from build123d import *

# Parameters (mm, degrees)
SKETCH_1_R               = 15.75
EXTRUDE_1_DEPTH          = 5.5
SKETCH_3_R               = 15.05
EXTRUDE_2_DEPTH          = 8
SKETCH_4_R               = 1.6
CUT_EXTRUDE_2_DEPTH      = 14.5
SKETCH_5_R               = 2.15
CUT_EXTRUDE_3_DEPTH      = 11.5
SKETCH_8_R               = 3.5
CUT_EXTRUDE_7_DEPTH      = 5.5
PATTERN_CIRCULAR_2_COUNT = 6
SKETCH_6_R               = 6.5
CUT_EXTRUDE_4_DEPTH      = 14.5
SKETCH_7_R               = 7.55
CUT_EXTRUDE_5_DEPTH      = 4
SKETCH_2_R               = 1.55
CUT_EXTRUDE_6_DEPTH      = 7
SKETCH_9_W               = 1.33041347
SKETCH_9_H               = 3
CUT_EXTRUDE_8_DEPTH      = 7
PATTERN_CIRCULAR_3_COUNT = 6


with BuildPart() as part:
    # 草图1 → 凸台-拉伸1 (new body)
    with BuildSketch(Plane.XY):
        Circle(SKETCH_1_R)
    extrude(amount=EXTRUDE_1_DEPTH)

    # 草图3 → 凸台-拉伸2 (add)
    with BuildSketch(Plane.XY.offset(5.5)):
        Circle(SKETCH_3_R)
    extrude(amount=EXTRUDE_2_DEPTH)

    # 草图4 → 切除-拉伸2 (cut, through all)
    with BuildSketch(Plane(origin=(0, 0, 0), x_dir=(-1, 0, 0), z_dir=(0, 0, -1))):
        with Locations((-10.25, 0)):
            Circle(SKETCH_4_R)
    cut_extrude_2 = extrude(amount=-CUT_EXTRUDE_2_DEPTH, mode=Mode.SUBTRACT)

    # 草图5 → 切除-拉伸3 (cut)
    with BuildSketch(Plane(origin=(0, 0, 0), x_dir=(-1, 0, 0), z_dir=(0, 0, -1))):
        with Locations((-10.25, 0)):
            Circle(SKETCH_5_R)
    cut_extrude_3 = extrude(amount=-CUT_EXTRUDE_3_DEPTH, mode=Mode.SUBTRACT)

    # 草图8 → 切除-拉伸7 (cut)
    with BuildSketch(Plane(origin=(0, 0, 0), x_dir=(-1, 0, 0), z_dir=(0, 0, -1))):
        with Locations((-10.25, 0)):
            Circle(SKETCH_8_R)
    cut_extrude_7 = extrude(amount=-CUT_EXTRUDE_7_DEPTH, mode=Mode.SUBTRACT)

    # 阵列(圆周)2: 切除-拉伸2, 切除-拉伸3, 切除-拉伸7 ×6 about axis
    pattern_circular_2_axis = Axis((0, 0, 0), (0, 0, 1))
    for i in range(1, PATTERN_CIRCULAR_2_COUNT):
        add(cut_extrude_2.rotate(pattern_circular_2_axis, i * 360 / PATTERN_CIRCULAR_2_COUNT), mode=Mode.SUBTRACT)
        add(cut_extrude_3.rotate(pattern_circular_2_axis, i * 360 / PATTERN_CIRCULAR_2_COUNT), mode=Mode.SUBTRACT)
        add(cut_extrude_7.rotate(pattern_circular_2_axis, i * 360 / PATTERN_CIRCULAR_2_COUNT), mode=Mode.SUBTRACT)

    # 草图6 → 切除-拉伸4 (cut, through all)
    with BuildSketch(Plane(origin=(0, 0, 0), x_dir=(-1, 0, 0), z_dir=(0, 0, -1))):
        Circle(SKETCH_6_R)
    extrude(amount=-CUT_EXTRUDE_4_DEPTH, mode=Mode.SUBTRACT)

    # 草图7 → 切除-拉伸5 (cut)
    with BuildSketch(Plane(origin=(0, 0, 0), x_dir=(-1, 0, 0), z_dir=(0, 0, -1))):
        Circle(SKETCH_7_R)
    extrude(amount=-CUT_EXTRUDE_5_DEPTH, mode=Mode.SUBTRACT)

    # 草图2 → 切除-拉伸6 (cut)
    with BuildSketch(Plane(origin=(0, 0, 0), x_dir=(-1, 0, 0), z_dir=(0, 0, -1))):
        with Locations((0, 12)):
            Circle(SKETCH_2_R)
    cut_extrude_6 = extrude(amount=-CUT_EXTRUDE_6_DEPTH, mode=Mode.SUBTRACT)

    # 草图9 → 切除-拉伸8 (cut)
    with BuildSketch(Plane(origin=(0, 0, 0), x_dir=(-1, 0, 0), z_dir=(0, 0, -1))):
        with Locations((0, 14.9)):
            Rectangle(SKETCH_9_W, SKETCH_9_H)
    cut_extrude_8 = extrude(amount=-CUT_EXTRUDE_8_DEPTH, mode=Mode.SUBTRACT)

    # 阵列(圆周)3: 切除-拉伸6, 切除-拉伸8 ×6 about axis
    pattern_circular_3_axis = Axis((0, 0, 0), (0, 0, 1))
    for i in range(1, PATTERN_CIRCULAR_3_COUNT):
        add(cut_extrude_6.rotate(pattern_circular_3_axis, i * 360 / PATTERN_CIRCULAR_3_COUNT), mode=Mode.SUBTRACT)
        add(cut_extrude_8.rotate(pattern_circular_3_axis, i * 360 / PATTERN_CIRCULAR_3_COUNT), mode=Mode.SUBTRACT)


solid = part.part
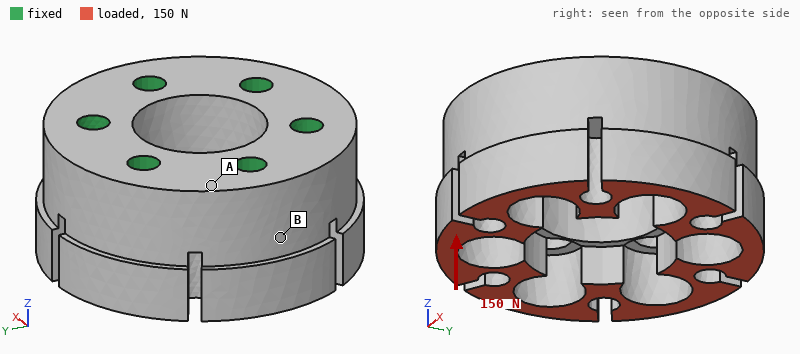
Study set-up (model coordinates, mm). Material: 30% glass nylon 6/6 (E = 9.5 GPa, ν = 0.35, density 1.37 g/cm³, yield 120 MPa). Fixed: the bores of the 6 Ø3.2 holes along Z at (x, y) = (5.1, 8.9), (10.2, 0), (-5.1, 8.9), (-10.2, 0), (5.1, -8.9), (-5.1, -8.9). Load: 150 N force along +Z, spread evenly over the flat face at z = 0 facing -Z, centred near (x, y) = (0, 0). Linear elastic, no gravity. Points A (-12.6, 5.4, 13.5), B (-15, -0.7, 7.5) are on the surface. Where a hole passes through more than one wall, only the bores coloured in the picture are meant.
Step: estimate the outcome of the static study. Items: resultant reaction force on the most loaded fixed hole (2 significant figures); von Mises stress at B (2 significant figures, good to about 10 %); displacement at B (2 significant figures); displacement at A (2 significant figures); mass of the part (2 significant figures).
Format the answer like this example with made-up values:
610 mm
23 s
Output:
25 N
0.77 MPa
1.2 µm
0.96 µm
7.8 g
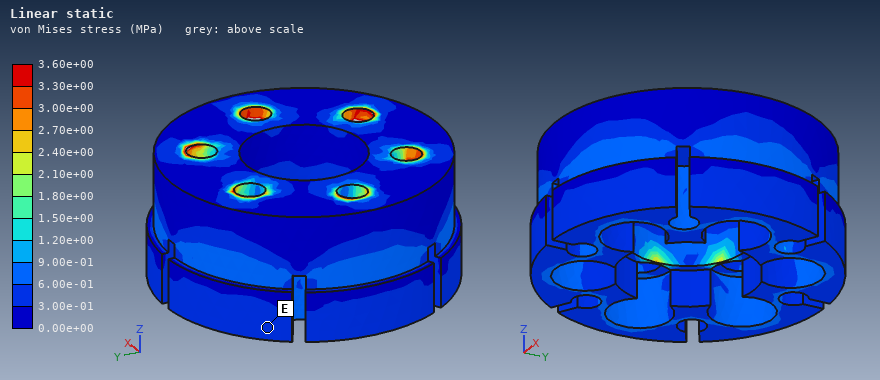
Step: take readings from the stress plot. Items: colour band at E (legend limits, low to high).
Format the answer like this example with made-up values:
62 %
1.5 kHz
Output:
3.00e-01 to 6.00e-01 MPa
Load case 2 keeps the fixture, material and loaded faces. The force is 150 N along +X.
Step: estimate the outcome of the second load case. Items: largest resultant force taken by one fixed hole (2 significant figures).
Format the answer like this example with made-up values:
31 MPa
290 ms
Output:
52 N
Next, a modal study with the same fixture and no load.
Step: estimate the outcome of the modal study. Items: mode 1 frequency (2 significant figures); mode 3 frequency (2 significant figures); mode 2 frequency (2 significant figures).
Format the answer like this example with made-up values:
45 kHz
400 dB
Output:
14 kHz
15 kHz
14 kHz
